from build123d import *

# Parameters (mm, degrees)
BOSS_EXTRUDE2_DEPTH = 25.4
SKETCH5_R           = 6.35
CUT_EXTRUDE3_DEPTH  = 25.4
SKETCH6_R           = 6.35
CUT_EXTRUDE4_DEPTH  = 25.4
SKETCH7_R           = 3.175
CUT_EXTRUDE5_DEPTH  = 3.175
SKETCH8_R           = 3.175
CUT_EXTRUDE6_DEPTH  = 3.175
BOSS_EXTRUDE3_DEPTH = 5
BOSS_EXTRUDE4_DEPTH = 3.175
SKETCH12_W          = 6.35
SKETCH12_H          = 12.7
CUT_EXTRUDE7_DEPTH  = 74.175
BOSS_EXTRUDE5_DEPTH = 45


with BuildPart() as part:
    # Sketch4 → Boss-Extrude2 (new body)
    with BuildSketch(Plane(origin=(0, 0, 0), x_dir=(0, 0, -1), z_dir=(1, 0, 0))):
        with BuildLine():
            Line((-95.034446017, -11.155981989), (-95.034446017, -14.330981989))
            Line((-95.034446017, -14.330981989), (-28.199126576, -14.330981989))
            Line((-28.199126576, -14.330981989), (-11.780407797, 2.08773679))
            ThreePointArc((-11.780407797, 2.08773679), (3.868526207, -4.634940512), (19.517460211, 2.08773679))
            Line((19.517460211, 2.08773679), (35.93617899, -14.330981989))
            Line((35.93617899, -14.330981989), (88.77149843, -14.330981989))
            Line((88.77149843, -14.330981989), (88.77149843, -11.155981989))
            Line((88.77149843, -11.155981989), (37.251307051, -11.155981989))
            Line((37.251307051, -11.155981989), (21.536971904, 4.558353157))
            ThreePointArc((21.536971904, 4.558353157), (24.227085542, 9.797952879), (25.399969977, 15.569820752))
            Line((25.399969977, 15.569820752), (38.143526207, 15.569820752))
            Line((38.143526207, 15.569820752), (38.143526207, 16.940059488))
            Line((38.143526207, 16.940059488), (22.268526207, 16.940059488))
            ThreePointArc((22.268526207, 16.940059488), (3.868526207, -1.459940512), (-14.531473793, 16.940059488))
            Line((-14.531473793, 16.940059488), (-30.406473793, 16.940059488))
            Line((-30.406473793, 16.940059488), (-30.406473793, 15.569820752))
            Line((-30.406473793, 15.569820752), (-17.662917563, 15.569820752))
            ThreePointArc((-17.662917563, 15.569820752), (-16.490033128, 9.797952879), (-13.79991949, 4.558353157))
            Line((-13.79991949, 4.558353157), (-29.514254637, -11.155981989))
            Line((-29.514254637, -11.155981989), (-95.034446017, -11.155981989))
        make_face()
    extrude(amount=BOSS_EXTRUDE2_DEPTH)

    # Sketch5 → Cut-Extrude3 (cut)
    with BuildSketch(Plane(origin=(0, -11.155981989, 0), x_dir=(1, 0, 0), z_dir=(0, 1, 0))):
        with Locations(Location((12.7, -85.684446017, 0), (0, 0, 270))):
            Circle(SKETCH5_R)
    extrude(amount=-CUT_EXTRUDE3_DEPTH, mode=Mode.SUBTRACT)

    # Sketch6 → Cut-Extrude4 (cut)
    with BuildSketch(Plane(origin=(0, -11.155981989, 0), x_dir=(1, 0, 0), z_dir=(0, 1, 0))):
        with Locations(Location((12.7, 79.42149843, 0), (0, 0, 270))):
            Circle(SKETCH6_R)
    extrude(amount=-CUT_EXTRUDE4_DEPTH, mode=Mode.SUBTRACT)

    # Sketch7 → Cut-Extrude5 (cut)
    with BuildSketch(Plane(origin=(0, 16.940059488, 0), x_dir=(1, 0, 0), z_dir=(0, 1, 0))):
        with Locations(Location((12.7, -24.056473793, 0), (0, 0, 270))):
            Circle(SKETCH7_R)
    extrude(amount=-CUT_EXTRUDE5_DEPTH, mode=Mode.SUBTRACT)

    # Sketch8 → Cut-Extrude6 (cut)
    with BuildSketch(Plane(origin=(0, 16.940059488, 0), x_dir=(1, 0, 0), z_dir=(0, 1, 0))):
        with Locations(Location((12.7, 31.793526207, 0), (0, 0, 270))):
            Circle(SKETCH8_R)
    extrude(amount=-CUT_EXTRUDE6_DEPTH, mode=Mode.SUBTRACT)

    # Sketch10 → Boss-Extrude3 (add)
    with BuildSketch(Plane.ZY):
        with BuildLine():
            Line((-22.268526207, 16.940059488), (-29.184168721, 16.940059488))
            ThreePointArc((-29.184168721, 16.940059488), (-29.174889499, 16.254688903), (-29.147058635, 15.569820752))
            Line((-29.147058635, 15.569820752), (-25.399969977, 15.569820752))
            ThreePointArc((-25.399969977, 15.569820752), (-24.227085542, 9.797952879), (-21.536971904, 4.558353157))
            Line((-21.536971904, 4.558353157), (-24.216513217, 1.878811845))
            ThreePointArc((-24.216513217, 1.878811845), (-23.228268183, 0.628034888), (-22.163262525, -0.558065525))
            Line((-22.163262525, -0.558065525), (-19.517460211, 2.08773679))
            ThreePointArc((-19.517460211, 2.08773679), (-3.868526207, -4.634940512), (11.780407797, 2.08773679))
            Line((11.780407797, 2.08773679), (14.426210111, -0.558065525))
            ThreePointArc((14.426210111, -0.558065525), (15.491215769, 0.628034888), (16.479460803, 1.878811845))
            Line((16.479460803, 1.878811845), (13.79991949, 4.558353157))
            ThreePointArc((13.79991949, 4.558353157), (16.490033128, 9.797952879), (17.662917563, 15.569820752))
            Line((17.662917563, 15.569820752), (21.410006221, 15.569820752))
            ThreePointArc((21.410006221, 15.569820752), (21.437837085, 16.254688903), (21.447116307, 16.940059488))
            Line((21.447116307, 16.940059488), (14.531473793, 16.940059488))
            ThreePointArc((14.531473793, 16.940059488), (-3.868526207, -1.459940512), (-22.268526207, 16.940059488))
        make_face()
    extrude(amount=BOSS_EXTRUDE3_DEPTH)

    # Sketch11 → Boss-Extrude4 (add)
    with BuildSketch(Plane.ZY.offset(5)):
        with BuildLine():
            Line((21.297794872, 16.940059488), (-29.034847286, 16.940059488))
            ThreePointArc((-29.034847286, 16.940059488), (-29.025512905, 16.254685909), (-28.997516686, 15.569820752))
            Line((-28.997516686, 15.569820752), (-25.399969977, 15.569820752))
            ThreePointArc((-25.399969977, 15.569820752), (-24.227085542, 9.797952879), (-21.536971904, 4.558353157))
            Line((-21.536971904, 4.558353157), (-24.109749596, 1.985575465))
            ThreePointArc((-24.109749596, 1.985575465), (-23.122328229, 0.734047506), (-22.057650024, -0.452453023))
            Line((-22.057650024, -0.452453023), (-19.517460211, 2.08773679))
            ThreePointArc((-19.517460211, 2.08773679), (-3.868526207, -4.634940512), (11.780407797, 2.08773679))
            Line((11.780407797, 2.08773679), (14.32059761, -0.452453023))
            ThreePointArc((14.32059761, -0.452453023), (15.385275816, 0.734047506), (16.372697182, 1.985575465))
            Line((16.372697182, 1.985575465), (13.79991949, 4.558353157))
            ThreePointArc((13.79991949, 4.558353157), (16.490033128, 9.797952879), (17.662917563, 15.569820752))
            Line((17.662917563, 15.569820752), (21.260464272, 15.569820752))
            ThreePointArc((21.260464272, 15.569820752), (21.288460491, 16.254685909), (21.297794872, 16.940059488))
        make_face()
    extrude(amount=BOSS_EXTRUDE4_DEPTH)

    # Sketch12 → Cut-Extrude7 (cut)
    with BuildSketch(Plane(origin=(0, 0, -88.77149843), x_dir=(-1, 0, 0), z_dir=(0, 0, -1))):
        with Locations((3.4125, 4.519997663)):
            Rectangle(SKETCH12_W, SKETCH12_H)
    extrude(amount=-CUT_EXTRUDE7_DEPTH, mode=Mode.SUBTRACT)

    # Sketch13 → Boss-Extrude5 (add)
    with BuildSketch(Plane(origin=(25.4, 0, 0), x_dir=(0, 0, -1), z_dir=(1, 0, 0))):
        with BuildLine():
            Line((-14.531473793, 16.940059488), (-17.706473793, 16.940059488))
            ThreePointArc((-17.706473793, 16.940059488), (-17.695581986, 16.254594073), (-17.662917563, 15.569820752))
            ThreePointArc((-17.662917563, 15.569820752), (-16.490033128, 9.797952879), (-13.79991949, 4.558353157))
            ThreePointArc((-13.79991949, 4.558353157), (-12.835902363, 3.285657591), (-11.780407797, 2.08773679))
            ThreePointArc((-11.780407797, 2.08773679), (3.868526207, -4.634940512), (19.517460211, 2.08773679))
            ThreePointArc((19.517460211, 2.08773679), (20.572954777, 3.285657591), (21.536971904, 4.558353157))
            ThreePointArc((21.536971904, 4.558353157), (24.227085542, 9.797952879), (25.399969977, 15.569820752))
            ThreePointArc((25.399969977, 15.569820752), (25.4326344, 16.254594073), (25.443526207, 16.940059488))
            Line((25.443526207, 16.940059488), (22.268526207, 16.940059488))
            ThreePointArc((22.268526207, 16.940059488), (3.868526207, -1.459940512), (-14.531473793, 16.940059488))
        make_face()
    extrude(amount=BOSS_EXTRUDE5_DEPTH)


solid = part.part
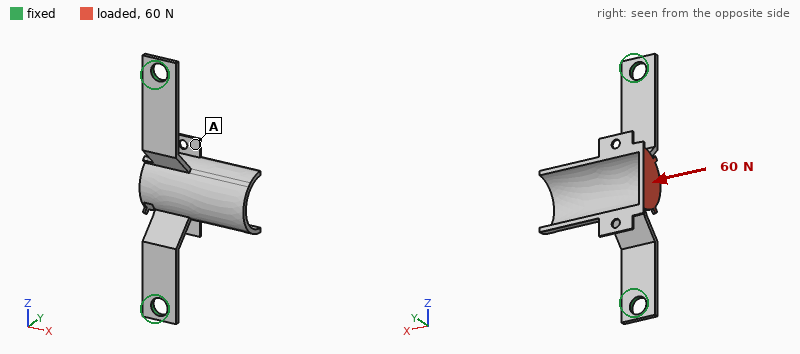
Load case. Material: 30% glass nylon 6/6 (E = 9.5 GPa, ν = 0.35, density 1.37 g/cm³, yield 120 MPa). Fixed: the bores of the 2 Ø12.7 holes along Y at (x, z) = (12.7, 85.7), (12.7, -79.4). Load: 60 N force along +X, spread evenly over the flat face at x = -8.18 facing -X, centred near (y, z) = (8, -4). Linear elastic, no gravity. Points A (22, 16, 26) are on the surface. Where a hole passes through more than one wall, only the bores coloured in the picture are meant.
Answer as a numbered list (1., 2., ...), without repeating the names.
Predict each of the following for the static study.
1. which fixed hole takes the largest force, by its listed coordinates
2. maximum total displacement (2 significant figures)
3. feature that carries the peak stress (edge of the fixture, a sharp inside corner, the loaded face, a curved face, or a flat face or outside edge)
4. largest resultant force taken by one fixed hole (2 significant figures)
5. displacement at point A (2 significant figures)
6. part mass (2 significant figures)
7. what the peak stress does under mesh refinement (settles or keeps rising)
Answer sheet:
1. (12.7, -79.4)
2. 1.8 mm
3. edge of the fixture
4. 35 N
5. 0.89 mm
6. 42 g
7. keeps rising
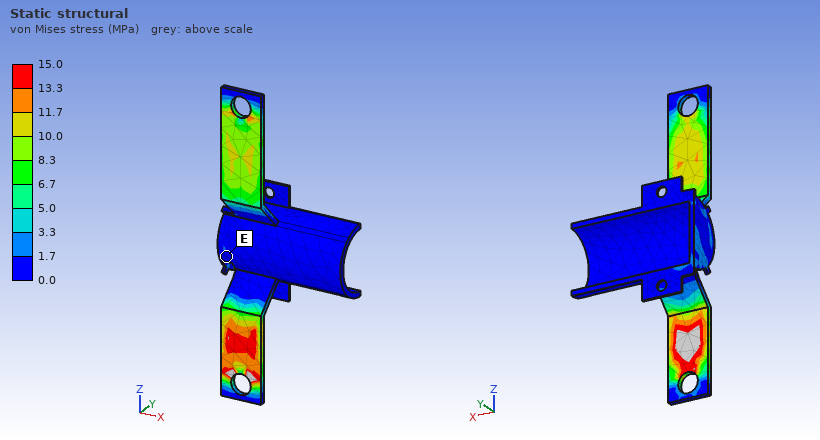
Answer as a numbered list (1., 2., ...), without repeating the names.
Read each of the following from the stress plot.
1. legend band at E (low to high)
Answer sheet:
1. 0.0 to 1.7 MPa
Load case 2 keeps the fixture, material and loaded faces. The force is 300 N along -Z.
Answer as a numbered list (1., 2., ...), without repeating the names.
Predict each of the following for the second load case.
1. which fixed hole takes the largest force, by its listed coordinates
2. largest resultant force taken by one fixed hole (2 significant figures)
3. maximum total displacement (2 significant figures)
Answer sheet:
1. (12.7, 85.7)
2. 190 N
3. 1.1 mm
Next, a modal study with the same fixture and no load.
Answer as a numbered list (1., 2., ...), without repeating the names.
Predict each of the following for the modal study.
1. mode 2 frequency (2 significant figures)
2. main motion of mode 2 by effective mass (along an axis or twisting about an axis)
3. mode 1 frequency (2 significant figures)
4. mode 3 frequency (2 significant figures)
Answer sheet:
1. 330 Hz
2. along Y
3. 190 Hz
4. 570 Hz
